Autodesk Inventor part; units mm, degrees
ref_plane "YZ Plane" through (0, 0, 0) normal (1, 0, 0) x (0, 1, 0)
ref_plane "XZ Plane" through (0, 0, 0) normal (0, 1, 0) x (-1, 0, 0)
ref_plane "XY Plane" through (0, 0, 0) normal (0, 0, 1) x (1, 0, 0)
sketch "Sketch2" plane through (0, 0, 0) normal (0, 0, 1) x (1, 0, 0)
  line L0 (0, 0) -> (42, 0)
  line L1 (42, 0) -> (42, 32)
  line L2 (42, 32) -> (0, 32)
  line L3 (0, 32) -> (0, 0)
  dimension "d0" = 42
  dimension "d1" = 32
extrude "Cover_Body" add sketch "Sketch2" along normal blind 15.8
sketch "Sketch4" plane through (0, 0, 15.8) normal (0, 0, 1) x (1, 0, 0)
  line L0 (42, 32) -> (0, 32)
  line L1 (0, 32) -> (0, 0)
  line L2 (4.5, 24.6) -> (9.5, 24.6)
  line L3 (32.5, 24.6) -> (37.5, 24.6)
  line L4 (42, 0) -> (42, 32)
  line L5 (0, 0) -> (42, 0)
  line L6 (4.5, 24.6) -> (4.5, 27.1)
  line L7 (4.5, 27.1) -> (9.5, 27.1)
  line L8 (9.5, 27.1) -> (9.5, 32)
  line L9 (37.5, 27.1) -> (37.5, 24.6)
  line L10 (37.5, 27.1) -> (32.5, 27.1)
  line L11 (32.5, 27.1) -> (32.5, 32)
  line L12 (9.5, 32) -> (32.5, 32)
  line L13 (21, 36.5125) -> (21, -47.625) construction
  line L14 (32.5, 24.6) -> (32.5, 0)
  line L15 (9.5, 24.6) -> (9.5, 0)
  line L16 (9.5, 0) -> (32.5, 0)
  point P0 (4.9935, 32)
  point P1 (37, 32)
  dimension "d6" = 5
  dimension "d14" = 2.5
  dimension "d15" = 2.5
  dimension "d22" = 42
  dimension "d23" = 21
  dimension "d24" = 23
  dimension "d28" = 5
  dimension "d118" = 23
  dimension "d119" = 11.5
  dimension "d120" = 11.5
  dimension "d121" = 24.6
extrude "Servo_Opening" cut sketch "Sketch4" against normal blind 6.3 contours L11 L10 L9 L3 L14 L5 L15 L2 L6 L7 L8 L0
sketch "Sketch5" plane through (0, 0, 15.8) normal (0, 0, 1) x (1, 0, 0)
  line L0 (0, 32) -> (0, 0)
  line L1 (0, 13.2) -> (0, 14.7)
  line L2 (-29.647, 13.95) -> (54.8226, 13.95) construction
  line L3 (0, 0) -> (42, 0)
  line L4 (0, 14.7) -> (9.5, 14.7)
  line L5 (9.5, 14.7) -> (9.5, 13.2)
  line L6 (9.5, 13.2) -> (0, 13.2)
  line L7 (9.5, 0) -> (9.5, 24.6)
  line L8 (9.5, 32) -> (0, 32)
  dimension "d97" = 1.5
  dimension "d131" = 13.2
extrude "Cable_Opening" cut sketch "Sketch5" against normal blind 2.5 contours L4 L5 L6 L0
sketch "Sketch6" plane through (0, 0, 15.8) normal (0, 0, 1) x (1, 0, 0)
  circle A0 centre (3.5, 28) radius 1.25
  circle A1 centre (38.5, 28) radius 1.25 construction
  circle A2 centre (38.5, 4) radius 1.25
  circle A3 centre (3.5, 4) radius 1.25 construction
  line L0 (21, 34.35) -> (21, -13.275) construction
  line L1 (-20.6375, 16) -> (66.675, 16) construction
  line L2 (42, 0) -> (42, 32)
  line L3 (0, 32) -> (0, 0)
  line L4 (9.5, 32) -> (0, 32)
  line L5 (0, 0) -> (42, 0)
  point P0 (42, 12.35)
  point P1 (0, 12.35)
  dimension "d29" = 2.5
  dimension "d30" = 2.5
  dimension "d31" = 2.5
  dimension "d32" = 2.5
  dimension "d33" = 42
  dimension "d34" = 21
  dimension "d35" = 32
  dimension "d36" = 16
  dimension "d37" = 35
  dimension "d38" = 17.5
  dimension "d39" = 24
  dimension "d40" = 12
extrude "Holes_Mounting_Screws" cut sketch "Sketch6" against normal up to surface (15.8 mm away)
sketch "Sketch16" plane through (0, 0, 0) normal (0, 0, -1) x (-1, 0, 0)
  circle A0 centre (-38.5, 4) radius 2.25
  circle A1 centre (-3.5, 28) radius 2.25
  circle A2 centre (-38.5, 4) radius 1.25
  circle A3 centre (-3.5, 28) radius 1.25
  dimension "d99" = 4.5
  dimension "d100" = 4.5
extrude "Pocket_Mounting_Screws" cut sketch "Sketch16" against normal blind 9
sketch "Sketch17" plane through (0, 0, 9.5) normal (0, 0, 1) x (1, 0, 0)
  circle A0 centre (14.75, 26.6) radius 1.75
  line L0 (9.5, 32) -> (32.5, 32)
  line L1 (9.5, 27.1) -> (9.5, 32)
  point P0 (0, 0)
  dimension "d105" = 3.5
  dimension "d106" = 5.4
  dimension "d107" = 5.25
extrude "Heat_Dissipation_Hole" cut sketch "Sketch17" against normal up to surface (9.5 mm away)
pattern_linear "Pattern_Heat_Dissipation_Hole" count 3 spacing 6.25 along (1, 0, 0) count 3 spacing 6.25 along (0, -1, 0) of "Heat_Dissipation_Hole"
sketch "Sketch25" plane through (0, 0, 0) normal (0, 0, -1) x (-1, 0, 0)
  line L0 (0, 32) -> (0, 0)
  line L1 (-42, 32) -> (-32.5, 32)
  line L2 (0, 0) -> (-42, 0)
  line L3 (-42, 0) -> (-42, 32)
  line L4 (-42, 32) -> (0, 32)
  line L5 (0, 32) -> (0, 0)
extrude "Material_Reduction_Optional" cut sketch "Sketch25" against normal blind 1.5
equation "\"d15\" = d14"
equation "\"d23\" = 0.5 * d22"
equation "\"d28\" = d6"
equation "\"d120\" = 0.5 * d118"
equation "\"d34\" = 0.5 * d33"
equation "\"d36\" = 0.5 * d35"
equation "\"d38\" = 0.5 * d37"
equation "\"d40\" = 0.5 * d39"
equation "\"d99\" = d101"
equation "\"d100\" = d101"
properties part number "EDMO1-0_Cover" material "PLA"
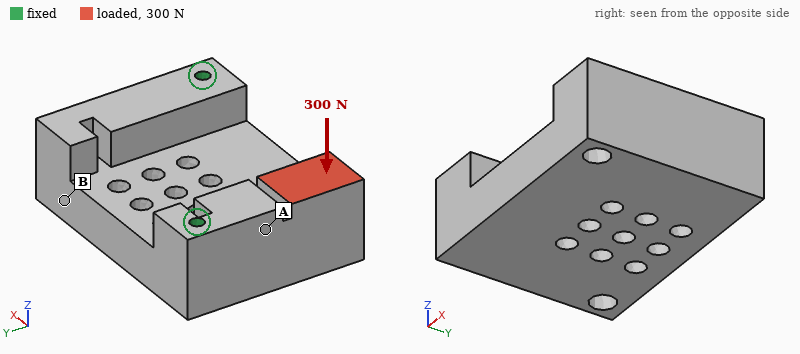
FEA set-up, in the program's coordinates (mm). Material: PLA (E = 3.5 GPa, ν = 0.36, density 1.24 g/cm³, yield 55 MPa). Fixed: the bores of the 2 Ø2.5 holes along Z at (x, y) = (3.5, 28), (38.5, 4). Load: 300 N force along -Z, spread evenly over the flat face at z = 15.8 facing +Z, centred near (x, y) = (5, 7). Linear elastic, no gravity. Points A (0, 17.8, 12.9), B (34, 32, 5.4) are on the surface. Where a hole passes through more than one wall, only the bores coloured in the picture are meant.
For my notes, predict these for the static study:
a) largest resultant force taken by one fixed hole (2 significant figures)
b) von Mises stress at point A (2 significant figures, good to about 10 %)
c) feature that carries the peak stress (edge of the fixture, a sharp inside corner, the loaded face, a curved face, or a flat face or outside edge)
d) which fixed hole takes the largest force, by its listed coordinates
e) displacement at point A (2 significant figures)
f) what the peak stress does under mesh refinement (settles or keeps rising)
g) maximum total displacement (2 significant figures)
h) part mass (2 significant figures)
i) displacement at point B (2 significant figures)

270 N
9.9 MPa
edge of the fixture
(3.5, 28)
0.17 mm
keeps rising
0.51 mm
17 g
0.18 mm
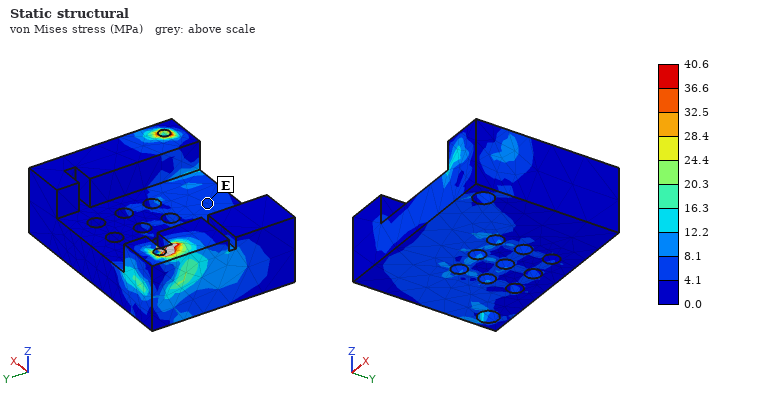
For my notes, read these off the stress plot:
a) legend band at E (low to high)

4.1 to 8.1 MPa
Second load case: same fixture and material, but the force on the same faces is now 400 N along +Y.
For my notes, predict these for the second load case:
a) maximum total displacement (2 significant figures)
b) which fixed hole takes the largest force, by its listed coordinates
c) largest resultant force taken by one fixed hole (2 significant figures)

0.21 mm
(3.5, 28)
390 N
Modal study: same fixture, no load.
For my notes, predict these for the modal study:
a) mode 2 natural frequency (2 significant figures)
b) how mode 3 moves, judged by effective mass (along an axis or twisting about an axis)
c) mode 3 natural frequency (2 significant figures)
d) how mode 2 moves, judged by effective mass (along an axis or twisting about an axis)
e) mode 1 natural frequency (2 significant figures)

3300 Hz
along X
5000 Hz
along Z
2000 Hz
